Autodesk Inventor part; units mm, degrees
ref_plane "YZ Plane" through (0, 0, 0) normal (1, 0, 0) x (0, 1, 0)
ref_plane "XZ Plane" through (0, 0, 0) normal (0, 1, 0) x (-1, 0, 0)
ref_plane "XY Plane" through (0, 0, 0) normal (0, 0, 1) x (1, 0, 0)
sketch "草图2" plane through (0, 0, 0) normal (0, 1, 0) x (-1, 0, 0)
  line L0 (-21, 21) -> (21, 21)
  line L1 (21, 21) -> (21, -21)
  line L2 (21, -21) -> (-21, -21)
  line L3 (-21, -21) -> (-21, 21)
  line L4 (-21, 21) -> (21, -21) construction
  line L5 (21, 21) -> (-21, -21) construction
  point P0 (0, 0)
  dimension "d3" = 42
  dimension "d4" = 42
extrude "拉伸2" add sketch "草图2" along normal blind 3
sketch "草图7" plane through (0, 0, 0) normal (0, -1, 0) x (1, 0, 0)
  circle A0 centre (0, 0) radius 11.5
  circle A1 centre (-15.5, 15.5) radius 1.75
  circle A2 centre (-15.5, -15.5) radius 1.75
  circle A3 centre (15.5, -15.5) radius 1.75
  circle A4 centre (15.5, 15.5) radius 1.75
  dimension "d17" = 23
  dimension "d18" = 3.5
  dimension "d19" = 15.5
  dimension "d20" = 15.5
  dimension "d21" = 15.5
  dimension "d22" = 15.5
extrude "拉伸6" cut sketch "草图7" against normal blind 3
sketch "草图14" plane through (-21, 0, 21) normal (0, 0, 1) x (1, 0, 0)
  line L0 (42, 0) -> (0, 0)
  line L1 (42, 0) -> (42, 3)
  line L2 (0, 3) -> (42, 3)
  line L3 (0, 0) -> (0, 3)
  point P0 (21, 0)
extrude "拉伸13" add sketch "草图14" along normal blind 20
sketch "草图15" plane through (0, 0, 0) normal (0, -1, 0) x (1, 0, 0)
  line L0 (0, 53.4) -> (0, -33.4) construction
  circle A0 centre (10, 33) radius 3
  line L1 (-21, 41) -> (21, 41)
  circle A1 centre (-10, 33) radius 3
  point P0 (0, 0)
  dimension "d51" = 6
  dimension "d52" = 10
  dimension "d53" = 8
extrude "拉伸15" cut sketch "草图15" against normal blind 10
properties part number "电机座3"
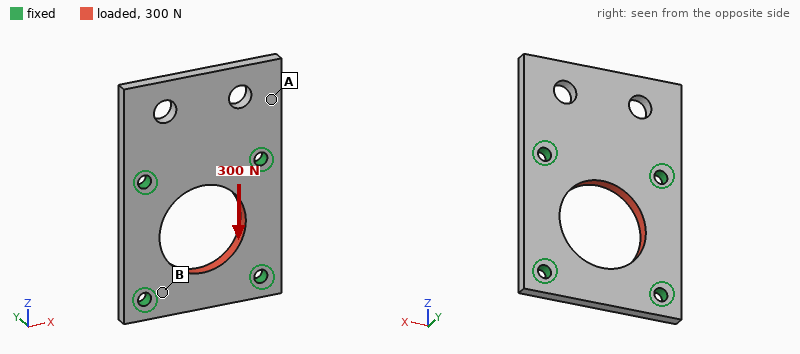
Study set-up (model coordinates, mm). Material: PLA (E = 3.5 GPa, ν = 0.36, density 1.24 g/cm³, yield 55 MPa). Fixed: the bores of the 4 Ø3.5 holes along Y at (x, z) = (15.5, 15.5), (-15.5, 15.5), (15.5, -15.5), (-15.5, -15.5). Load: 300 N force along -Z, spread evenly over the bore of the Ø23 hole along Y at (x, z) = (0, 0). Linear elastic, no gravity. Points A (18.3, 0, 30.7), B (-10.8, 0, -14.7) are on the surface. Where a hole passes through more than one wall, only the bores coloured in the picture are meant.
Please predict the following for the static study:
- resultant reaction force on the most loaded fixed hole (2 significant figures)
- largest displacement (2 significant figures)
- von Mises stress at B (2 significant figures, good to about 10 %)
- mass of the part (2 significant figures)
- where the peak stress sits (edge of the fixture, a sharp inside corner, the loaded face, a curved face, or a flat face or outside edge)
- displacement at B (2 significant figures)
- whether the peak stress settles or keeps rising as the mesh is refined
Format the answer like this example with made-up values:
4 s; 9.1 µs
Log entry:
78 N; 20 µm; 2.3 MPa; 7.8 g; edge of the fixture; 6.8 µm; keeps rising
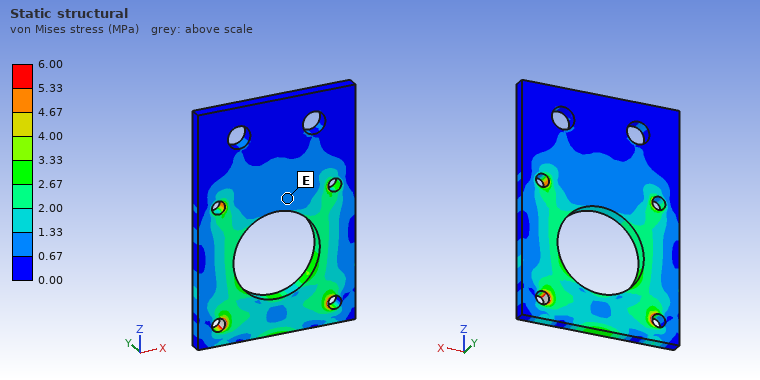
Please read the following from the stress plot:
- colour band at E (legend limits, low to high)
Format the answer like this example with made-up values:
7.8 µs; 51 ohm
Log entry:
0.67 to 1.33 MPa
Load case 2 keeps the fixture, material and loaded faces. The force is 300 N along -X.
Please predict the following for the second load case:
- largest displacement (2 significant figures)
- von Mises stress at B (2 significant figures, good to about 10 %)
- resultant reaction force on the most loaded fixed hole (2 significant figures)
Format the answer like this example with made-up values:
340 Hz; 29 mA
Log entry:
18 µm; 2.4 MPa; 78 N
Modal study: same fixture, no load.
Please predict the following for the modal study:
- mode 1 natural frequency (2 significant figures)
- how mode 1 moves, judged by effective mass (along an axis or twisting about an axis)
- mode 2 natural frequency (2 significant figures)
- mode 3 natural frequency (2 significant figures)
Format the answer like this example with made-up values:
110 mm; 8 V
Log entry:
1200 Hz; along Y; 2200 Hz; 4000 Hz
